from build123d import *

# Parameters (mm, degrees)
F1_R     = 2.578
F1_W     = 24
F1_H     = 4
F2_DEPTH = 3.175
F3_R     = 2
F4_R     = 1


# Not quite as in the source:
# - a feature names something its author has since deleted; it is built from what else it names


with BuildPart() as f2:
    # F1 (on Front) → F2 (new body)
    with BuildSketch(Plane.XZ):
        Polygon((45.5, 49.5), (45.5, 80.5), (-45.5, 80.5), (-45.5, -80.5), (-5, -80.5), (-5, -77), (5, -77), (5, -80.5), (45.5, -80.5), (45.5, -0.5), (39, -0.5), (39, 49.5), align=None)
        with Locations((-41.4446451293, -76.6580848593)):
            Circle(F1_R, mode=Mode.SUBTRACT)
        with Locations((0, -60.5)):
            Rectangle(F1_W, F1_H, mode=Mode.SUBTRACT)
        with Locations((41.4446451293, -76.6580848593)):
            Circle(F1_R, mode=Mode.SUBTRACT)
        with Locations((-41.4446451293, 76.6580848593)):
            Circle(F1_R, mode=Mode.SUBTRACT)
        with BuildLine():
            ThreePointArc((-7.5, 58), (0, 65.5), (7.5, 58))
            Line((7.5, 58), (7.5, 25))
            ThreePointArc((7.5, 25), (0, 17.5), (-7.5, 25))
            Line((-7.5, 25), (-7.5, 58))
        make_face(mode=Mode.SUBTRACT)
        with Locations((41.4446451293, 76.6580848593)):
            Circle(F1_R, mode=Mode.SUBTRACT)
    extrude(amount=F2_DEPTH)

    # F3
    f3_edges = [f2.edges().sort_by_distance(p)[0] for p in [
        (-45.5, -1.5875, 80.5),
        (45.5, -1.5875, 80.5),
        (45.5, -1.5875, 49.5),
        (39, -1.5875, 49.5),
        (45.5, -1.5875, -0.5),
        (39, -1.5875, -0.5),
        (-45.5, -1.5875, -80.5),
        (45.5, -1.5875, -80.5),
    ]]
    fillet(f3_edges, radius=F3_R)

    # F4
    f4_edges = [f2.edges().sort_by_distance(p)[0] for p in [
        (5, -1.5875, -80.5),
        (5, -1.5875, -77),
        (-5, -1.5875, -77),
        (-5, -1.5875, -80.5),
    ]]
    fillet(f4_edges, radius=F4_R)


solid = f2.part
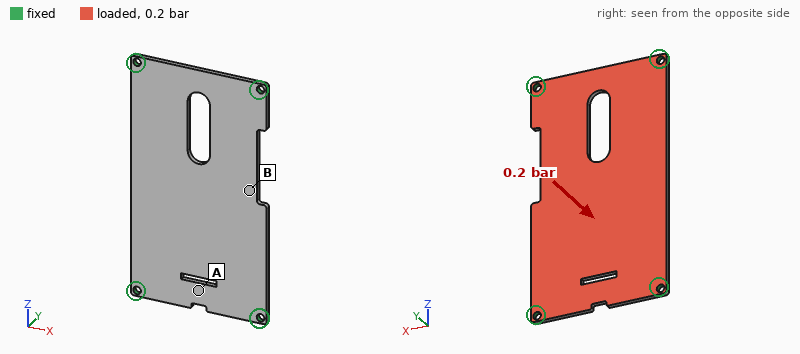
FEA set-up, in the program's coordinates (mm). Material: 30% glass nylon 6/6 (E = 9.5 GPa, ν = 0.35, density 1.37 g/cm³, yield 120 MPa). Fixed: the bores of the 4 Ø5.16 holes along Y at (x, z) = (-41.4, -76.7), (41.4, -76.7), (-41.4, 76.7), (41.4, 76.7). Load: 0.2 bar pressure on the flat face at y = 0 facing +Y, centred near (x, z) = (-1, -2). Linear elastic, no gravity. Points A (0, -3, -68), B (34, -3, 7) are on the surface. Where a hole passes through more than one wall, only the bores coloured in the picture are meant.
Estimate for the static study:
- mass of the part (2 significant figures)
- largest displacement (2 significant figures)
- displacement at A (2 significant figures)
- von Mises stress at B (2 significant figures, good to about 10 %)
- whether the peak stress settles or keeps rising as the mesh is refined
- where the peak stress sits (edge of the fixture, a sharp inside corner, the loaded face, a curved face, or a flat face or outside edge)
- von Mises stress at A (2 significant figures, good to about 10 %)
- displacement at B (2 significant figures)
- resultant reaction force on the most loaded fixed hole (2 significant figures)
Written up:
58 g
1.7 mm
0.35 mm
17 MPa
keeps rising
edge of the fixture
6.0 MPa
1.6 mm
70 N
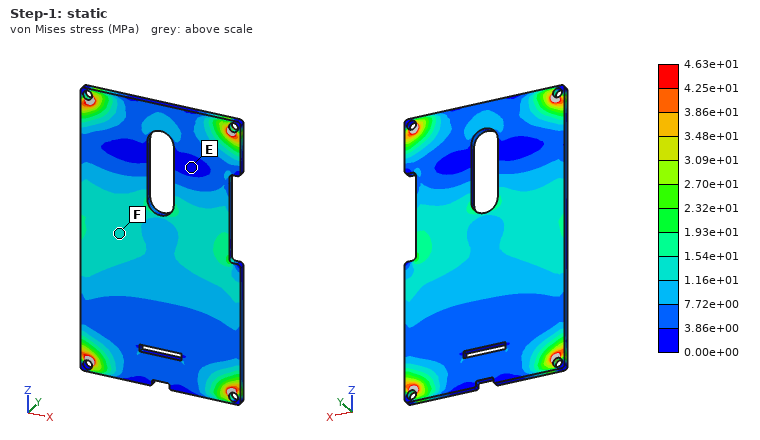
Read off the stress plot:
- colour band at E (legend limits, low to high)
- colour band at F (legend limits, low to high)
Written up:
0.00e+00 to 3.86e+00 MPa
1.16e+01 to 1.54e+01 MPa
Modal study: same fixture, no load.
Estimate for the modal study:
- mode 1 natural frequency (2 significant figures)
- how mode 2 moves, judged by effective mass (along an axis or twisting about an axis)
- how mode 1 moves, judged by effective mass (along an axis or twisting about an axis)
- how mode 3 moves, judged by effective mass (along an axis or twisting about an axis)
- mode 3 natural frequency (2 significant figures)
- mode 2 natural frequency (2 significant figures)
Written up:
300 Hz
twisting about Z
along Y
twisting about X
810 Hz
540 Hz
